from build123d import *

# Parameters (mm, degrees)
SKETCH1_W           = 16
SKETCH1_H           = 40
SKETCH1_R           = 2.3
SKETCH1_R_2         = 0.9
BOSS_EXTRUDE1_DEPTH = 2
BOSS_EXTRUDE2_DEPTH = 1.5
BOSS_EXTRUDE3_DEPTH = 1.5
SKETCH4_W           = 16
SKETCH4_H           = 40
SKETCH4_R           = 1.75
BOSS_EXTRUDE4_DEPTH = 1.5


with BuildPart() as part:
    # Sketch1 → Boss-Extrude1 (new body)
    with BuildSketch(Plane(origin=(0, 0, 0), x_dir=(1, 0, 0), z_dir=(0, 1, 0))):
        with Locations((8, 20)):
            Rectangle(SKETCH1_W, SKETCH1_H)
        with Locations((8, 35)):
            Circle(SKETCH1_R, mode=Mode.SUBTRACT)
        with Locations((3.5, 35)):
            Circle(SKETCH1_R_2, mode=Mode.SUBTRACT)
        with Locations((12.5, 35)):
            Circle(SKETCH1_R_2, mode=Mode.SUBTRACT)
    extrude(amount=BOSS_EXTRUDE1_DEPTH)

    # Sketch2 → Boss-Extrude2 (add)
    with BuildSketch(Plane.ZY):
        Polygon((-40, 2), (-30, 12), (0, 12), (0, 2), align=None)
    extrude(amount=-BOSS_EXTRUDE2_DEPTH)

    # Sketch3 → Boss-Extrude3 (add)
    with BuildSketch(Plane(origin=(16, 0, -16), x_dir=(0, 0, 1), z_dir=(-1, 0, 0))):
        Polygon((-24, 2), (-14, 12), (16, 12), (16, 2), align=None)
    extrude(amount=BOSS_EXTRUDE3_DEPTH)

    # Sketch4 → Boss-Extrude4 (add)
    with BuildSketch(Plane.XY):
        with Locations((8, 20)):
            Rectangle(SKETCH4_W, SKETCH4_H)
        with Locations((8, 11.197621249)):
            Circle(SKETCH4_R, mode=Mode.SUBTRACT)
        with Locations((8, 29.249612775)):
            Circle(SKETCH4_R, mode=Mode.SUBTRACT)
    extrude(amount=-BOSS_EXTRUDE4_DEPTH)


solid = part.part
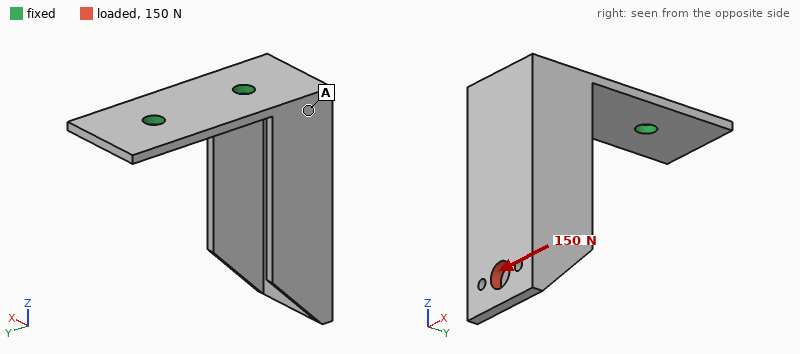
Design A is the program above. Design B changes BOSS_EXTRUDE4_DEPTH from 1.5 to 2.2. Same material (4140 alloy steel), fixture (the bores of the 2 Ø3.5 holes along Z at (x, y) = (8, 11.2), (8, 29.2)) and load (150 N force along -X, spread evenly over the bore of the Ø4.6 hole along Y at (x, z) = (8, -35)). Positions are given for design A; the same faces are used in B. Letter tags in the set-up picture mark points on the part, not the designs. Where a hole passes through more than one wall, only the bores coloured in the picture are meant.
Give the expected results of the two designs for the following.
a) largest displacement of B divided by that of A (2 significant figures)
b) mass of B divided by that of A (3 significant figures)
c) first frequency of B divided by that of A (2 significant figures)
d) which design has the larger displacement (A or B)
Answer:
0.50
1.13
1.5
A
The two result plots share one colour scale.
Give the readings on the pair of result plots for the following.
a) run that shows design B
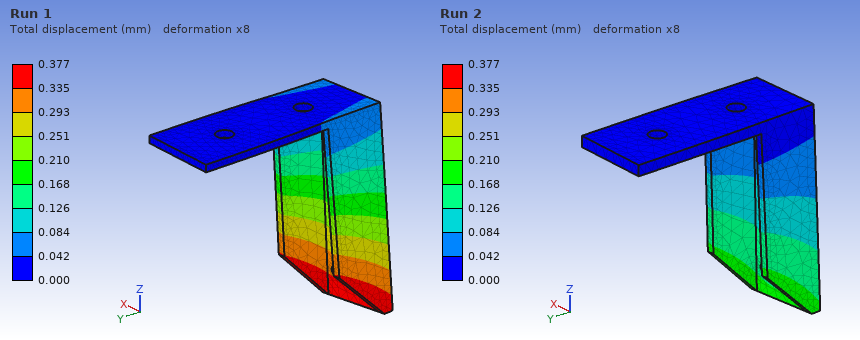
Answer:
Run 2
